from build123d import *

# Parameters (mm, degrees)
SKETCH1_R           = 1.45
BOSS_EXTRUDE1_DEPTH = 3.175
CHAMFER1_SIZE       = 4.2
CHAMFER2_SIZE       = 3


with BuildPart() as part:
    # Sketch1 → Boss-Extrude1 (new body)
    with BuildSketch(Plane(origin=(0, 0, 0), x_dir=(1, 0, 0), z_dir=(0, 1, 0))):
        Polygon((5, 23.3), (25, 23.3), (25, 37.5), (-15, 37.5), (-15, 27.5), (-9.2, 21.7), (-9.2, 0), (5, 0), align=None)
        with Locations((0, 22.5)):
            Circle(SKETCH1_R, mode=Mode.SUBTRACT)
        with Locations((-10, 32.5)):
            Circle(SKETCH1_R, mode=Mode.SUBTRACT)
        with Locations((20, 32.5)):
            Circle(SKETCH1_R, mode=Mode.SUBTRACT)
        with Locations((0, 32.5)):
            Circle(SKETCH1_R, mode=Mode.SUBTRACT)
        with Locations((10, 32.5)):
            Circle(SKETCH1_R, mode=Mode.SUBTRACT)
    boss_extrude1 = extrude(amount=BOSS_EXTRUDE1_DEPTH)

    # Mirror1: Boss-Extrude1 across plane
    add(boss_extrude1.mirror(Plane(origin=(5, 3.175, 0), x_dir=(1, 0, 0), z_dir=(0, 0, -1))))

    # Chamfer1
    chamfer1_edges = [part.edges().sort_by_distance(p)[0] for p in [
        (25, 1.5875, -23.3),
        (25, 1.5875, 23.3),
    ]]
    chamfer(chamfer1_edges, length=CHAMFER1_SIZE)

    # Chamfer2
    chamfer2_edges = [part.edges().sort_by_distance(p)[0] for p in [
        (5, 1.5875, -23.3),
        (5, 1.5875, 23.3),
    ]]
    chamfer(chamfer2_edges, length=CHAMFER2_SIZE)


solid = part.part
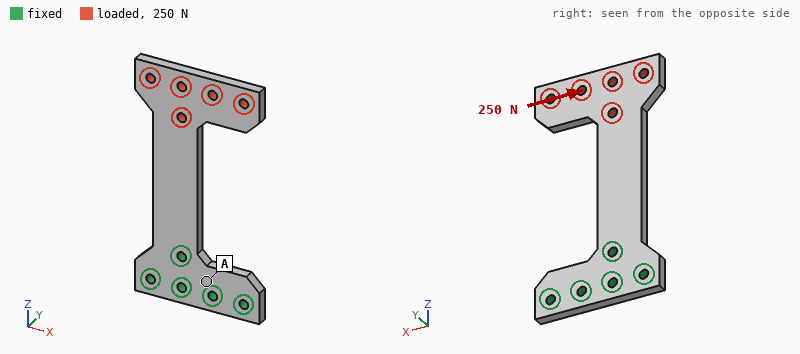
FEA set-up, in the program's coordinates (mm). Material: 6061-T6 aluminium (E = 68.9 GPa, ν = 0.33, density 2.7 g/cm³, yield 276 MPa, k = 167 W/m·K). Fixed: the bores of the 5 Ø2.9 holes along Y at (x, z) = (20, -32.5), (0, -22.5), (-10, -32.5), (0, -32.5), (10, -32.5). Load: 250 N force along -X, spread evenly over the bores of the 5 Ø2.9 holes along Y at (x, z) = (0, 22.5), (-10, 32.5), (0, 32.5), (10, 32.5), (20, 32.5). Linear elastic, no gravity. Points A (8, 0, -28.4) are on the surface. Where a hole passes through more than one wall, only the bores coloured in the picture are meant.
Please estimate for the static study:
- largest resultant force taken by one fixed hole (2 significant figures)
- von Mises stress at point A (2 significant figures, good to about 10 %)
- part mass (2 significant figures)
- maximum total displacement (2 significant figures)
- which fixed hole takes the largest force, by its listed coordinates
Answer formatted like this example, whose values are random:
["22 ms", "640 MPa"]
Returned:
["740 N", "18 MPa", "15 g", "0.39 mm", "(-10, -32.5)"]
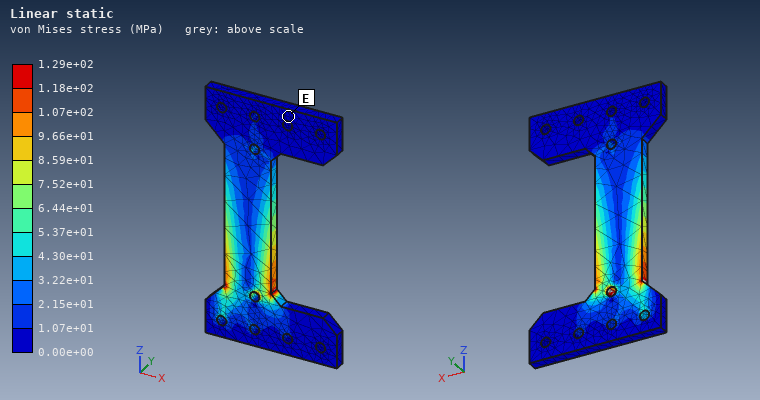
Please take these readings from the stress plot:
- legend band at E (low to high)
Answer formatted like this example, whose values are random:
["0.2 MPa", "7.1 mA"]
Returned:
["0.00e+00 to 1.07e+01 MPa"]
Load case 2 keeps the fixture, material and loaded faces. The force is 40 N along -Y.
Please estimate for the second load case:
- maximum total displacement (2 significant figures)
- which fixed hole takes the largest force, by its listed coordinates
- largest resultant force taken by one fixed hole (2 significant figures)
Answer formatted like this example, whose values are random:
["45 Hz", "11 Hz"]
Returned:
["0.98 mm", "(0, -22.5)", "140 N"]
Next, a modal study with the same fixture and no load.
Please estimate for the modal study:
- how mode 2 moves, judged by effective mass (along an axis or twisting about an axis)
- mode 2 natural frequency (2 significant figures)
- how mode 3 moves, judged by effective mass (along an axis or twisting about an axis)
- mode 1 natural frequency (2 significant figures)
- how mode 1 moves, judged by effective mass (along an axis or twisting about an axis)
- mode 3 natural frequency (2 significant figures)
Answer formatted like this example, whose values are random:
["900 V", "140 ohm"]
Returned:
["twisting about Z", "1600 Hz", "along X", "500 Hz", "along Y", "1900 Hz"]
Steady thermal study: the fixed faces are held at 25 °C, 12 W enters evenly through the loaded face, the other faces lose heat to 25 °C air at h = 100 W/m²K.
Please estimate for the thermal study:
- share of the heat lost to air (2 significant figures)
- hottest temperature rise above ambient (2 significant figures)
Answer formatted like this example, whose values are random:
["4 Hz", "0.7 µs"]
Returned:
["62 %", "41 K"]
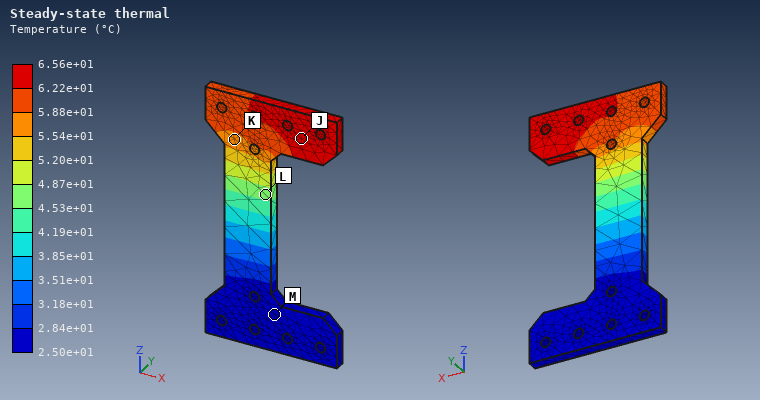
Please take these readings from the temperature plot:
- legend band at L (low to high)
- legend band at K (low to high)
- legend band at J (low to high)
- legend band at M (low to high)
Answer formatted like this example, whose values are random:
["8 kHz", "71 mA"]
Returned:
["4.53e+01 to 4.87e+01 °C", "5.54e+01 to 5.88e+01 °C", "6.22e+01 to 6.56e+01 °C", "2.50e+01 to 2.84e+01 °C"]
